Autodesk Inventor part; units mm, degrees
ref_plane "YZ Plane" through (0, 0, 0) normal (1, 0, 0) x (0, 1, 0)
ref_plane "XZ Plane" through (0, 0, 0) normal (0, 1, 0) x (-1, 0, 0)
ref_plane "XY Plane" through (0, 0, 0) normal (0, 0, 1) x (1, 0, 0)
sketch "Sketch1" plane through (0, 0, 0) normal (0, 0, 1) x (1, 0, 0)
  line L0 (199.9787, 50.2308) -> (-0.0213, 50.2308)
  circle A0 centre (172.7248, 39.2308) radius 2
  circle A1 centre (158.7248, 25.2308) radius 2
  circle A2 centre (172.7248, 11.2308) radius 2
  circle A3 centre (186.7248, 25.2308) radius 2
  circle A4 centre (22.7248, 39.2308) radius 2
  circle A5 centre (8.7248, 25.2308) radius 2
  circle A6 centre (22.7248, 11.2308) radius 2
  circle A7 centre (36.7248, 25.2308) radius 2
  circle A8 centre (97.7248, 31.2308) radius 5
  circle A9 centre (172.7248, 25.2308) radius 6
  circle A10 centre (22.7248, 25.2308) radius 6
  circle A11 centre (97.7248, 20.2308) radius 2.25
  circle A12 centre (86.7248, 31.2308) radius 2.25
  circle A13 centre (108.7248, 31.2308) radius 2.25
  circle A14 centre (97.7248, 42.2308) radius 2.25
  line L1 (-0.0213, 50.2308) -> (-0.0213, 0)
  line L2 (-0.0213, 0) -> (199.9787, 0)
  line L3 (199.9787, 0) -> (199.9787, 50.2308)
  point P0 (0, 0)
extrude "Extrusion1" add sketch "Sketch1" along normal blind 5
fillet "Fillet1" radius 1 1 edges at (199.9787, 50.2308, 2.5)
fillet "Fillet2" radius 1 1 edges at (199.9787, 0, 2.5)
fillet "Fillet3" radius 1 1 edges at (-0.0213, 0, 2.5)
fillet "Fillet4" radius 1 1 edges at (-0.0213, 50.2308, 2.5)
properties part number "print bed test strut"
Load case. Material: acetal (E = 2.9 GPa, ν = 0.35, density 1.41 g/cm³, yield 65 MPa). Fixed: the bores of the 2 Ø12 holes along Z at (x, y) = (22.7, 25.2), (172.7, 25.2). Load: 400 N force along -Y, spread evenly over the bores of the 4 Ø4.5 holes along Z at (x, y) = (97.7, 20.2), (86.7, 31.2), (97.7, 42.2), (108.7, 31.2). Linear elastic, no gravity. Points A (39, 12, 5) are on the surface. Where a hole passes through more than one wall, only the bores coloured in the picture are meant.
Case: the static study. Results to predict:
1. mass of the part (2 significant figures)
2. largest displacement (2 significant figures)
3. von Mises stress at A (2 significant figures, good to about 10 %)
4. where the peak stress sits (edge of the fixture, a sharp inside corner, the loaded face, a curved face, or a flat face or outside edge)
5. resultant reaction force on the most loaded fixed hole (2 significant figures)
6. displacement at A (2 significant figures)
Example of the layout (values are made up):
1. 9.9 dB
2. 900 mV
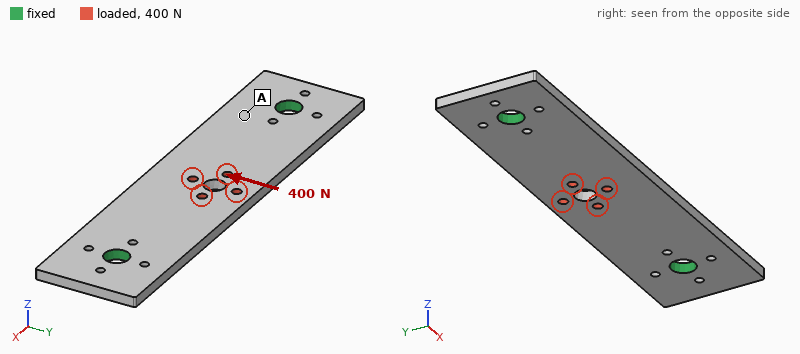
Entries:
1. 68 g
2. 0.17 mm
3. 1.5 MPa
4. edge of the fixture
5. 200 N
6. 0.044 mm
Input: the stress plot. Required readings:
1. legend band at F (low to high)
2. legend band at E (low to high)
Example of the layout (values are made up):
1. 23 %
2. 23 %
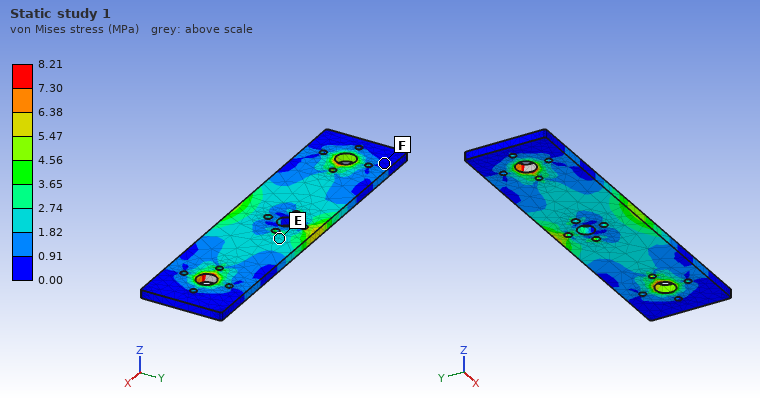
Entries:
1. 0.00 to 0.91 MPa
2. 1.82 to 2.74 MPa
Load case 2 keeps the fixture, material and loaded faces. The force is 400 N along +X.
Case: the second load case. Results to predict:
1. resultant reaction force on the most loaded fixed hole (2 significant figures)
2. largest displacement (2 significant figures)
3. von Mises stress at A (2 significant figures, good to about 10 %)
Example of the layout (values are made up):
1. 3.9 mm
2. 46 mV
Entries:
1. 200 N
2. 28 µm
3. 0.70 MPa
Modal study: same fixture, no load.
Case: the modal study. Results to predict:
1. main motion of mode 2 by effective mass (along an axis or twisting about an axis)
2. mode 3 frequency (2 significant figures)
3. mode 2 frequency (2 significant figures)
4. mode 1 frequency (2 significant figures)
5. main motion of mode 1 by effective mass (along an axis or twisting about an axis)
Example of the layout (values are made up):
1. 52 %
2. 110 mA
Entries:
1. twisting about X
2. 920 Hz
3. 610 Hz
4. 340 Hz
5. along Z
